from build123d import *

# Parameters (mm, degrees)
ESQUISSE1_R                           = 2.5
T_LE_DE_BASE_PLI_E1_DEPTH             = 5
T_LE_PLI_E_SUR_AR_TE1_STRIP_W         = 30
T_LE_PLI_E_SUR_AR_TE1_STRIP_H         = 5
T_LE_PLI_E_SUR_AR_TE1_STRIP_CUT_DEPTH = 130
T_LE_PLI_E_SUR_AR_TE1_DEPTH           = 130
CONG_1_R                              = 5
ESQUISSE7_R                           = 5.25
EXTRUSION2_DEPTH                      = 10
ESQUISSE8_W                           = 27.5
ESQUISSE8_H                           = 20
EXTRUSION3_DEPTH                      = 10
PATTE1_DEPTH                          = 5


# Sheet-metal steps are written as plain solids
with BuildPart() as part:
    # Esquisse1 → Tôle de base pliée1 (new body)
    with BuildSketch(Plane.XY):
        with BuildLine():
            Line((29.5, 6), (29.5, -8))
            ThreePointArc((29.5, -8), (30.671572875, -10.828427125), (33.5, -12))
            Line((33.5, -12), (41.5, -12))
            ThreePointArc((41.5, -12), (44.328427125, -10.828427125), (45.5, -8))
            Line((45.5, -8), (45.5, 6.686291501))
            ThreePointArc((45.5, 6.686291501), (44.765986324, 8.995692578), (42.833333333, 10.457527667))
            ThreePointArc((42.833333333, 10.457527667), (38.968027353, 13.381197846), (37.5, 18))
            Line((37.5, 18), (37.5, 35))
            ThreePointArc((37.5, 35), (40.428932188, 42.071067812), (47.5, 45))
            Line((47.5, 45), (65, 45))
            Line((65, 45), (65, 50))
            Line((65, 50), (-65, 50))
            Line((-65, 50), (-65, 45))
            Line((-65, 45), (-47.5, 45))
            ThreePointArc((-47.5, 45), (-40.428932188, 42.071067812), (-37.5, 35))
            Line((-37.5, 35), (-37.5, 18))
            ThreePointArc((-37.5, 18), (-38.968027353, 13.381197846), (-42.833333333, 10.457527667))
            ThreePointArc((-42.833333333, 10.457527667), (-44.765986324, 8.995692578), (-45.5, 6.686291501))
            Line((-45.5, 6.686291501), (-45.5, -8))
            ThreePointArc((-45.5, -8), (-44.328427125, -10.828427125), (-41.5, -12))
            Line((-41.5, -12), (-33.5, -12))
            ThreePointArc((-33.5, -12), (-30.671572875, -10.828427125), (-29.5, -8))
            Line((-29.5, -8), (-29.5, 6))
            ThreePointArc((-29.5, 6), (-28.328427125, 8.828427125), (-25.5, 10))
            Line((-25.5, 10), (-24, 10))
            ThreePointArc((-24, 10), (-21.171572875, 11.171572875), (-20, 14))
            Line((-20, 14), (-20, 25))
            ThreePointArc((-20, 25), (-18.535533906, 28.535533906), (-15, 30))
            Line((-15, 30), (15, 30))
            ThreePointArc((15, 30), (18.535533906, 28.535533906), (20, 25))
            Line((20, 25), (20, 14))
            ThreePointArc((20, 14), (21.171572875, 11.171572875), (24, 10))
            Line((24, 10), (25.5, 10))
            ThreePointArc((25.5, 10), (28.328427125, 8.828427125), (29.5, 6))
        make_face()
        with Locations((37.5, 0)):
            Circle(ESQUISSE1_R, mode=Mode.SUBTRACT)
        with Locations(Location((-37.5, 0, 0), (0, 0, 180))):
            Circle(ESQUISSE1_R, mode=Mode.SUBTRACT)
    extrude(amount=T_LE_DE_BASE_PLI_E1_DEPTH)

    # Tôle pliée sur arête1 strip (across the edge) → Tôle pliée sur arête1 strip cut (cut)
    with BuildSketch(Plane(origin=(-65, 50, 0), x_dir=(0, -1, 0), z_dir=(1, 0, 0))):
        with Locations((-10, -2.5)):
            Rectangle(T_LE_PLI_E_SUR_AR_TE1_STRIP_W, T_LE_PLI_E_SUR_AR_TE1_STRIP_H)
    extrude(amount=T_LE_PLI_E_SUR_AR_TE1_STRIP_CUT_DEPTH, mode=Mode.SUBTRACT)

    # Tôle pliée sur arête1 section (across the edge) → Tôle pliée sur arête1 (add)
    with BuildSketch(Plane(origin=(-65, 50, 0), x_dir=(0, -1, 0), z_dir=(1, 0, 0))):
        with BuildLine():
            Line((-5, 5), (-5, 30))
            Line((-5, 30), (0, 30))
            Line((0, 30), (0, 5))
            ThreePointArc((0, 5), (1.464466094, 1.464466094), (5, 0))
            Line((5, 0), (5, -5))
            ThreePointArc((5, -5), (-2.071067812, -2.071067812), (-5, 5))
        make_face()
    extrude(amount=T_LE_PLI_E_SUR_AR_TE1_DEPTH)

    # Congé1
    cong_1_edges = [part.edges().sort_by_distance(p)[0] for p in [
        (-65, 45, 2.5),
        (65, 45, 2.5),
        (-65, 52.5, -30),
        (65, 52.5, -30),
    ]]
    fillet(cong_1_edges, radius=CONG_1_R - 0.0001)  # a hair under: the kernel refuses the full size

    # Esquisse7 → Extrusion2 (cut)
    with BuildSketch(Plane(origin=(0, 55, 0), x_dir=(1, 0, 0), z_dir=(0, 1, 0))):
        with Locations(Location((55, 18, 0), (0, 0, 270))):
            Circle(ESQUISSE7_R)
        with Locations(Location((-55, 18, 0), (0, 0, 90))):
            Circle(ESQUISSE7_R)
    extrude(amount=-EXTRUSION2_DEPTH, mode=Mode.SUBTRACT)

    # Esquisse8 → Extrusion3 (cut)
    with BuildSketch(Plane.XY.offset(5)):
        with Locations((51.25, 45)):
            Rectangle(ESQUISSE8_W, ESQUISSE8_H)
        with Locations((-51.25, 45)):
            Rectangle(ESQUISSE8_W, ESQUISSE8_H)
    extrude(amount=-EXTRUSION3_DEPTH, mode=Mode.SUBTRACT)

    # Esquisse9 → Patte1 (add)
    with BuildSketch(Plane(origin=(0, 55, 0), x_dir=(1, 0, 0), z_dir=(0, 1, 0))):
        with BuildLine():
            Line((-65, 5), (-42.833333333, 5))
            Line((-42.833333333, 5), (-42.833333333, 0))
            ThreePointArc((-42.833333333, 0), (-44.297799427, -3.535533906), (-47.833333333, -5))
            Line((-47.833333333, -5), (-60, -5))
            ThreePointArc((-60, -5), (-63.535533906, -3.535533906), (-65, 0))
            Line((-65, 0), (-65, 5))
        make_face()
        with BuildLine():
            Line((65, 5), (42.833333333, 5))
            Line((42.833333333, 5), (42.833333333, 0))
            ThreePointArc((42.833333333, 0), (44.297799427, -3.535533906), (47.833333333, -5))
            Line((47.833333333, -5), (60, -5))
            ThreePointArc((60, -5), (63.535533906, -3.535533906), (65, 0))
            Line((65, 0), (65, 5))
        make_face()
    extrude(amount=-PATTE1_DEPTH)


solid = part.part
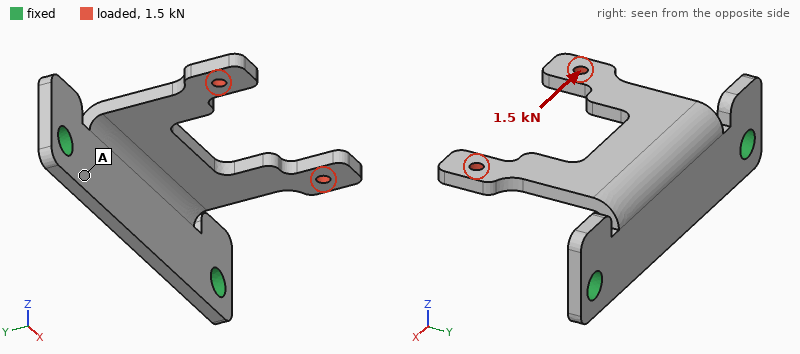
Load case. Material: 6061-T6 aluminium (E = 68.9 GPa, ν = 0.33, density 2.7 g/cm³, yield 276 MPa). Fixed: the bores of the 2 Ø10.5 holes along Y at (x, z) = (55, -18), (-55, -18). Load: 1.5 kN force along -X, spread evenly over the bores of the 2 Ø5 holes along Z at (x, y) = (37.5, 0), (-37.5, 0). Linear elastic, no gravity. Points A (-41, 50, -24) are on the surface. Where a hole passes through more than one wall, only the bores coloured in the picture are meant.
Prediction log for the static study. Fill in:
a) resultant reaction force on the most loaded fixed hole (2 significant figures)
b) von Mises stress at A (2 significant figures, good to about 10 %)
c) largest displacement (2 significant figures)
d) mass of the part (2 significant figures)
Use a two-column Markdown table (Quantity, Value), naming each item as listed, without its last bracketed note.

| Quantity | Value |
|---|---|
| resultant reaction force on the most loaded fixed hole | 1.3 kN |
| von Mises stress at A | 34 MPa |
| largest displacement | 0.68 mm |
| mass of the part | 93 g |
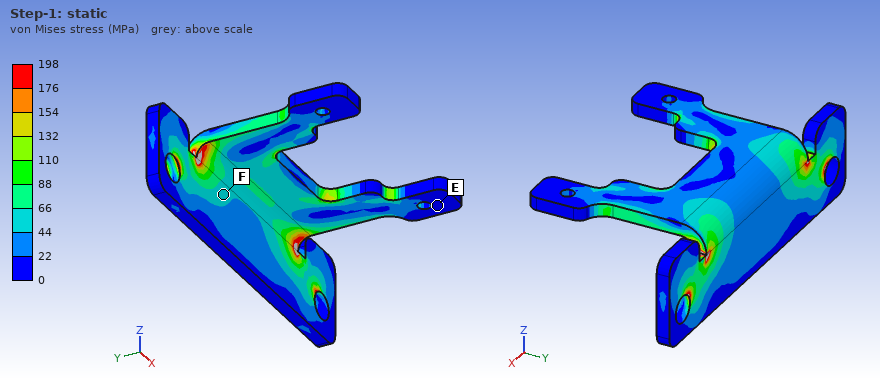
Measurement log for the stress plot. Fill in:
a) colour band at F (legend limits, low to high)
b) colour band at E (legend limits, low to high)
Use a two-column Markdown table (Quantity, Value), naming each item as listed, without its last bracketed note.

| Quantity | Value |
|---|---|
| colour band at F | 44 to 66 MPa |
| colour band at E | 0 to 22 MPa |
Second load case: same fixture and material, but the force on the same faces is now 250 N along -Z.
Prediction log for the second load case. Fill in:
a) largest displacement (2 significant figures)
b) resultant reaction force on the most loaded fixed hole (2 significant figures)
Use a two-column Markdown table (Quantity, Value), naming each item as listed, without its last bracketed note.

| Quantity | Value |
|---|---|
| largest displacement | 1.0 mm |
| resultant reaction force on the most loaded fixed hole | 130 N |
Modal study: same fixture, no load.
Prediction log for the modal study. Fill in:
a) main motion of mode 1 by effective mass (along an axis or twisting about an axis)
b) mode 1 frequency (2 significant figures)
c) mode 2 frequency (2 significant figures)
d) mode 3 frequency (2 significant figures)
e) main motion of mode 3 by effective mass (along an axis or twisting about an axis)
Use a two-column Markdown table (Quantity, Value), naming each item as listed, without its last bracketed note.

| Quantity | Value |
|---|---|
| main motion of mode 1 by effective mass | along Z |
| mode 1 frequency | 770 Hz |
| mode 2 frequency | 1100 Hz |
| mode 3 frequency | 2200 Hz |
| main motion of mode 3 by effective mass | along Y |
